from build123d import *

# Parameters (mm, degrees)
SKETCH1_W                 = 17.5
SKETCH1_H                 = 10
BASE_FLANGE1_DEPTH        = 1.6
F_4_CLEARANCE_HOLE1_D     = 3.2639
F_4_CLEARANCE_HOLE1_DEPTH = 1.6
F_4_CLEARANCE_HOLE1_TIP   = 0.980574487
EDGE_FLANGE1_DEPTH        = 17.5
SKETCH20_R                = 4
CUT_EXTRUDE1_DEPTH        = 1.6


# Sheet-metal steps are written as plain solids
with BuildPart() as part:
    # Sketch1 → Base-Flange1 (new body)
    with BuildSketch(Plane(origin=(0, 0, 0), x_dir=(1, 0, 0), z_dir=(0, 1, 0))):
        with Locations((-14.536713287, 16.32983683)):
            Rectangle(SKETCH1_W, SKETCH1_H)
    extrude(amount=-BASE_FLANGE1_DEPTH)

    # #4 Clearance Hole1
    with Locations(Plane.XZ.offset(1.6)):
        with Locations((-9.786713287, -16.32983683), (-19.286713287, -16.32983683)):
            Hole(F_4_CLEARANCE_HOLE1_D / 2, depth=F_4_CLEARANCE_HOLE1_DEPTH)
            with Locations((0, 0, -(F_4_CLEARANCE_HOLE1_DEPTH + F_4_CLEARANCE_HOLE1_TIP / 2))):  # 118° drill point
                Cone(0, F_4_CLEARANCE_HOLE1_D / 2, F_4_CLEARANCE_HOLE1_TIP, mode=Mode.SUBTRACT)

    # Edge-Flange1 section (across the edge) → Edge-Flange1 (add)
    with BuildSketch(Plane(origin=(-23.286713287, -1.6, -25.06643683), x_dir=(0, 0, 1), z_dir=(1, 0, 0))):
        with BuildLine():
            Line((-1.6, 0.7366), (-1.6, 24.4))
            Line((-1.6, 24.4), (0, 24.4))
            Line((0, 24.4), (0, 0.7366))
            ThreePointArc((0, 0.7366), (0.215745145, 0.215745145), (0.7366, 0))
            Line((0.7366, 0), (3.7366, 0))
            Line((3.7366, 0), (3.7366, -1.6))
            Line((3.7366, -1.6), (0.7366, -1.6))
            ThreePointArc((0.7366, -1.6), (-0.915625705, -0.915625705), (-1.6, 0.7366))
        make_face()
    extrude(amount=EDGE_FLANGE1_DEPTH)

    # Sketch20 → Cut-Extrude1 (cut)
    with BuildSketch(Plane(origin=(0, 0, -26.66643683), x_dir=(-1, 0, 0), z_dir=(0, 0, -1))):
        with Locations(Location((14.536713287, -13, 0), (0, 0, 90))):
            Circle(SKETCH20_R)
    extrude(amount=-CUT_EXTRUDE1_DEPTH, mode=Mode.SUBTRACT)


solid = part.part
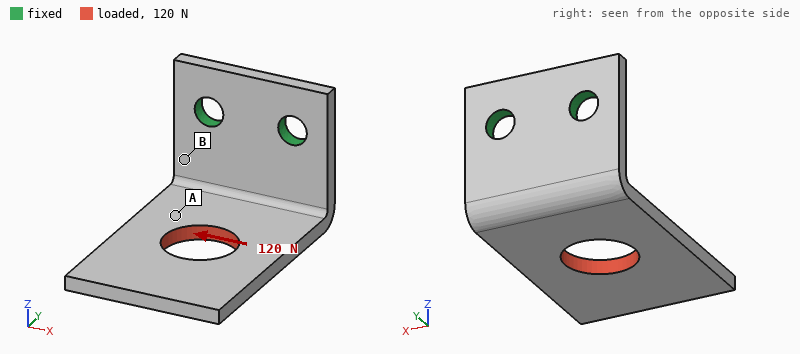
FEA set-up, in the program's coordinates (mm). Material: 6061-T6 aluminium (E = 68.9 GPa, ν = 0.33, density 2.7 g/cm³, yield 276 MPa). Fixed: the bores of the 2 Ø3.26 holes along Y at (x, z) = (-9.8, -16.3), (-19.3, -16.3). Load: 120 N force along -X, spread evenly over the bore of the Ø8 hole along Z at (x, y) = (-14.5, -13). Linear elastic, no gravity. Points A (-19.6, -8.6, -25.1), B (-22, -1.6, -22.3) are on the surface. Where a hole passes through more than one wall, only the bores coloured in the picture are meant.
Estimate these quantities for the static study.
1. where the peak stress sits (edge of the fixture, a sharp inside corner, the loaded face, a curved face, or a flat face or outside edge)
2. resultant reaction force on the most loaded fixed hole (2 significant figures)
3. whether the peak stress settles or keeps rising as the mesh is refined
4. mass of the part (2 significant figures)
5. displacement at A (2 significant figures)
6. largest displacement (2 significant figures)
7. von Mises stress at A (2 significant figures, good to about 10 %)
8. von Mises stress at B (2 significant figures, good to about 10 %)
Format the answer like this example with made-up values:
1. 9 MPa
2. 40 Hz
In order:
1. edge of the fixture
2. 160 N
3. keeps rising
4. 2.7 g
5. 0.086 mm
6. 0.24 mm
7. 21 MPa
8. 79 MPa
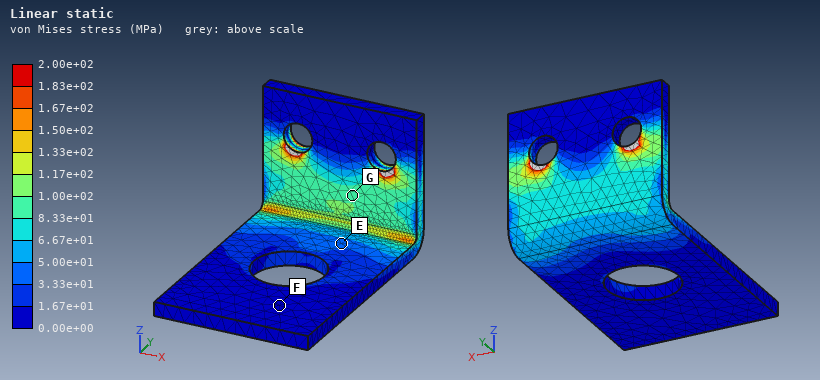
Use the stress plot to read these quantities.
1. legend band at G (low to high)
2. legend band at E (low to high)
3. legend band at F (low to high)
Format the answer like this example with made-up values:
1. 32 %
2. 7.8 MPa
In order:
1. 8.33e+01 to 1.00e+02 MPa
2. 3.33e+01 to 5.00e+01 MPa
3. 0.00e+00 to 1.67e+01 MPa
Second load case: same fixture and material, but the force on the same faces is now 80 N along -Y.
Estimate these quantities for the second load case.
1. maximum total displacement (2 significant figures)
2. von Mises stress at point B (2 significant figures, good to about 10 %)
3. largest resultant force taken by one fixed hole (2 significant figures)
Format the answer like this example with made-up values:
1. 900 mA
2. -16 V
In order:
1. 0.17 mm
2. 37 MPa
3. 40 N
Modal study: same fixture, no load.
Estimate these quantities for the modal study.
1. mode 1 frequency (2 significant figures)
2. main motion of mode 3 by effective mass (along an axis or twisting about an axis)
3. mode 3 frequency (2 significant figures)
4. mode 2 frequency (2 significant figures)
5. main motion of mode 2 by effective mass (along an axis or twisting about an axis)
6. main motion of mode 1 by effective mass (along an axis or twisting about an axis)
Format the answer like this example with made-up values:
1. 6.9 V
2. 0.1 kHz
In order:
1. 1400 Hz
2. twisting about Y
3. 5800 Hz
4. 3100 Hz
5. along X
6. along Z
